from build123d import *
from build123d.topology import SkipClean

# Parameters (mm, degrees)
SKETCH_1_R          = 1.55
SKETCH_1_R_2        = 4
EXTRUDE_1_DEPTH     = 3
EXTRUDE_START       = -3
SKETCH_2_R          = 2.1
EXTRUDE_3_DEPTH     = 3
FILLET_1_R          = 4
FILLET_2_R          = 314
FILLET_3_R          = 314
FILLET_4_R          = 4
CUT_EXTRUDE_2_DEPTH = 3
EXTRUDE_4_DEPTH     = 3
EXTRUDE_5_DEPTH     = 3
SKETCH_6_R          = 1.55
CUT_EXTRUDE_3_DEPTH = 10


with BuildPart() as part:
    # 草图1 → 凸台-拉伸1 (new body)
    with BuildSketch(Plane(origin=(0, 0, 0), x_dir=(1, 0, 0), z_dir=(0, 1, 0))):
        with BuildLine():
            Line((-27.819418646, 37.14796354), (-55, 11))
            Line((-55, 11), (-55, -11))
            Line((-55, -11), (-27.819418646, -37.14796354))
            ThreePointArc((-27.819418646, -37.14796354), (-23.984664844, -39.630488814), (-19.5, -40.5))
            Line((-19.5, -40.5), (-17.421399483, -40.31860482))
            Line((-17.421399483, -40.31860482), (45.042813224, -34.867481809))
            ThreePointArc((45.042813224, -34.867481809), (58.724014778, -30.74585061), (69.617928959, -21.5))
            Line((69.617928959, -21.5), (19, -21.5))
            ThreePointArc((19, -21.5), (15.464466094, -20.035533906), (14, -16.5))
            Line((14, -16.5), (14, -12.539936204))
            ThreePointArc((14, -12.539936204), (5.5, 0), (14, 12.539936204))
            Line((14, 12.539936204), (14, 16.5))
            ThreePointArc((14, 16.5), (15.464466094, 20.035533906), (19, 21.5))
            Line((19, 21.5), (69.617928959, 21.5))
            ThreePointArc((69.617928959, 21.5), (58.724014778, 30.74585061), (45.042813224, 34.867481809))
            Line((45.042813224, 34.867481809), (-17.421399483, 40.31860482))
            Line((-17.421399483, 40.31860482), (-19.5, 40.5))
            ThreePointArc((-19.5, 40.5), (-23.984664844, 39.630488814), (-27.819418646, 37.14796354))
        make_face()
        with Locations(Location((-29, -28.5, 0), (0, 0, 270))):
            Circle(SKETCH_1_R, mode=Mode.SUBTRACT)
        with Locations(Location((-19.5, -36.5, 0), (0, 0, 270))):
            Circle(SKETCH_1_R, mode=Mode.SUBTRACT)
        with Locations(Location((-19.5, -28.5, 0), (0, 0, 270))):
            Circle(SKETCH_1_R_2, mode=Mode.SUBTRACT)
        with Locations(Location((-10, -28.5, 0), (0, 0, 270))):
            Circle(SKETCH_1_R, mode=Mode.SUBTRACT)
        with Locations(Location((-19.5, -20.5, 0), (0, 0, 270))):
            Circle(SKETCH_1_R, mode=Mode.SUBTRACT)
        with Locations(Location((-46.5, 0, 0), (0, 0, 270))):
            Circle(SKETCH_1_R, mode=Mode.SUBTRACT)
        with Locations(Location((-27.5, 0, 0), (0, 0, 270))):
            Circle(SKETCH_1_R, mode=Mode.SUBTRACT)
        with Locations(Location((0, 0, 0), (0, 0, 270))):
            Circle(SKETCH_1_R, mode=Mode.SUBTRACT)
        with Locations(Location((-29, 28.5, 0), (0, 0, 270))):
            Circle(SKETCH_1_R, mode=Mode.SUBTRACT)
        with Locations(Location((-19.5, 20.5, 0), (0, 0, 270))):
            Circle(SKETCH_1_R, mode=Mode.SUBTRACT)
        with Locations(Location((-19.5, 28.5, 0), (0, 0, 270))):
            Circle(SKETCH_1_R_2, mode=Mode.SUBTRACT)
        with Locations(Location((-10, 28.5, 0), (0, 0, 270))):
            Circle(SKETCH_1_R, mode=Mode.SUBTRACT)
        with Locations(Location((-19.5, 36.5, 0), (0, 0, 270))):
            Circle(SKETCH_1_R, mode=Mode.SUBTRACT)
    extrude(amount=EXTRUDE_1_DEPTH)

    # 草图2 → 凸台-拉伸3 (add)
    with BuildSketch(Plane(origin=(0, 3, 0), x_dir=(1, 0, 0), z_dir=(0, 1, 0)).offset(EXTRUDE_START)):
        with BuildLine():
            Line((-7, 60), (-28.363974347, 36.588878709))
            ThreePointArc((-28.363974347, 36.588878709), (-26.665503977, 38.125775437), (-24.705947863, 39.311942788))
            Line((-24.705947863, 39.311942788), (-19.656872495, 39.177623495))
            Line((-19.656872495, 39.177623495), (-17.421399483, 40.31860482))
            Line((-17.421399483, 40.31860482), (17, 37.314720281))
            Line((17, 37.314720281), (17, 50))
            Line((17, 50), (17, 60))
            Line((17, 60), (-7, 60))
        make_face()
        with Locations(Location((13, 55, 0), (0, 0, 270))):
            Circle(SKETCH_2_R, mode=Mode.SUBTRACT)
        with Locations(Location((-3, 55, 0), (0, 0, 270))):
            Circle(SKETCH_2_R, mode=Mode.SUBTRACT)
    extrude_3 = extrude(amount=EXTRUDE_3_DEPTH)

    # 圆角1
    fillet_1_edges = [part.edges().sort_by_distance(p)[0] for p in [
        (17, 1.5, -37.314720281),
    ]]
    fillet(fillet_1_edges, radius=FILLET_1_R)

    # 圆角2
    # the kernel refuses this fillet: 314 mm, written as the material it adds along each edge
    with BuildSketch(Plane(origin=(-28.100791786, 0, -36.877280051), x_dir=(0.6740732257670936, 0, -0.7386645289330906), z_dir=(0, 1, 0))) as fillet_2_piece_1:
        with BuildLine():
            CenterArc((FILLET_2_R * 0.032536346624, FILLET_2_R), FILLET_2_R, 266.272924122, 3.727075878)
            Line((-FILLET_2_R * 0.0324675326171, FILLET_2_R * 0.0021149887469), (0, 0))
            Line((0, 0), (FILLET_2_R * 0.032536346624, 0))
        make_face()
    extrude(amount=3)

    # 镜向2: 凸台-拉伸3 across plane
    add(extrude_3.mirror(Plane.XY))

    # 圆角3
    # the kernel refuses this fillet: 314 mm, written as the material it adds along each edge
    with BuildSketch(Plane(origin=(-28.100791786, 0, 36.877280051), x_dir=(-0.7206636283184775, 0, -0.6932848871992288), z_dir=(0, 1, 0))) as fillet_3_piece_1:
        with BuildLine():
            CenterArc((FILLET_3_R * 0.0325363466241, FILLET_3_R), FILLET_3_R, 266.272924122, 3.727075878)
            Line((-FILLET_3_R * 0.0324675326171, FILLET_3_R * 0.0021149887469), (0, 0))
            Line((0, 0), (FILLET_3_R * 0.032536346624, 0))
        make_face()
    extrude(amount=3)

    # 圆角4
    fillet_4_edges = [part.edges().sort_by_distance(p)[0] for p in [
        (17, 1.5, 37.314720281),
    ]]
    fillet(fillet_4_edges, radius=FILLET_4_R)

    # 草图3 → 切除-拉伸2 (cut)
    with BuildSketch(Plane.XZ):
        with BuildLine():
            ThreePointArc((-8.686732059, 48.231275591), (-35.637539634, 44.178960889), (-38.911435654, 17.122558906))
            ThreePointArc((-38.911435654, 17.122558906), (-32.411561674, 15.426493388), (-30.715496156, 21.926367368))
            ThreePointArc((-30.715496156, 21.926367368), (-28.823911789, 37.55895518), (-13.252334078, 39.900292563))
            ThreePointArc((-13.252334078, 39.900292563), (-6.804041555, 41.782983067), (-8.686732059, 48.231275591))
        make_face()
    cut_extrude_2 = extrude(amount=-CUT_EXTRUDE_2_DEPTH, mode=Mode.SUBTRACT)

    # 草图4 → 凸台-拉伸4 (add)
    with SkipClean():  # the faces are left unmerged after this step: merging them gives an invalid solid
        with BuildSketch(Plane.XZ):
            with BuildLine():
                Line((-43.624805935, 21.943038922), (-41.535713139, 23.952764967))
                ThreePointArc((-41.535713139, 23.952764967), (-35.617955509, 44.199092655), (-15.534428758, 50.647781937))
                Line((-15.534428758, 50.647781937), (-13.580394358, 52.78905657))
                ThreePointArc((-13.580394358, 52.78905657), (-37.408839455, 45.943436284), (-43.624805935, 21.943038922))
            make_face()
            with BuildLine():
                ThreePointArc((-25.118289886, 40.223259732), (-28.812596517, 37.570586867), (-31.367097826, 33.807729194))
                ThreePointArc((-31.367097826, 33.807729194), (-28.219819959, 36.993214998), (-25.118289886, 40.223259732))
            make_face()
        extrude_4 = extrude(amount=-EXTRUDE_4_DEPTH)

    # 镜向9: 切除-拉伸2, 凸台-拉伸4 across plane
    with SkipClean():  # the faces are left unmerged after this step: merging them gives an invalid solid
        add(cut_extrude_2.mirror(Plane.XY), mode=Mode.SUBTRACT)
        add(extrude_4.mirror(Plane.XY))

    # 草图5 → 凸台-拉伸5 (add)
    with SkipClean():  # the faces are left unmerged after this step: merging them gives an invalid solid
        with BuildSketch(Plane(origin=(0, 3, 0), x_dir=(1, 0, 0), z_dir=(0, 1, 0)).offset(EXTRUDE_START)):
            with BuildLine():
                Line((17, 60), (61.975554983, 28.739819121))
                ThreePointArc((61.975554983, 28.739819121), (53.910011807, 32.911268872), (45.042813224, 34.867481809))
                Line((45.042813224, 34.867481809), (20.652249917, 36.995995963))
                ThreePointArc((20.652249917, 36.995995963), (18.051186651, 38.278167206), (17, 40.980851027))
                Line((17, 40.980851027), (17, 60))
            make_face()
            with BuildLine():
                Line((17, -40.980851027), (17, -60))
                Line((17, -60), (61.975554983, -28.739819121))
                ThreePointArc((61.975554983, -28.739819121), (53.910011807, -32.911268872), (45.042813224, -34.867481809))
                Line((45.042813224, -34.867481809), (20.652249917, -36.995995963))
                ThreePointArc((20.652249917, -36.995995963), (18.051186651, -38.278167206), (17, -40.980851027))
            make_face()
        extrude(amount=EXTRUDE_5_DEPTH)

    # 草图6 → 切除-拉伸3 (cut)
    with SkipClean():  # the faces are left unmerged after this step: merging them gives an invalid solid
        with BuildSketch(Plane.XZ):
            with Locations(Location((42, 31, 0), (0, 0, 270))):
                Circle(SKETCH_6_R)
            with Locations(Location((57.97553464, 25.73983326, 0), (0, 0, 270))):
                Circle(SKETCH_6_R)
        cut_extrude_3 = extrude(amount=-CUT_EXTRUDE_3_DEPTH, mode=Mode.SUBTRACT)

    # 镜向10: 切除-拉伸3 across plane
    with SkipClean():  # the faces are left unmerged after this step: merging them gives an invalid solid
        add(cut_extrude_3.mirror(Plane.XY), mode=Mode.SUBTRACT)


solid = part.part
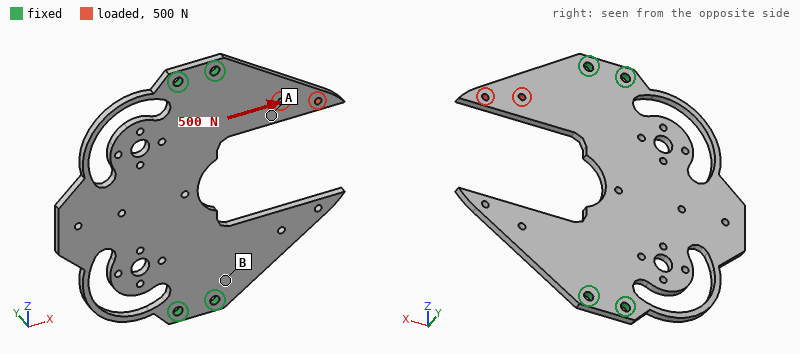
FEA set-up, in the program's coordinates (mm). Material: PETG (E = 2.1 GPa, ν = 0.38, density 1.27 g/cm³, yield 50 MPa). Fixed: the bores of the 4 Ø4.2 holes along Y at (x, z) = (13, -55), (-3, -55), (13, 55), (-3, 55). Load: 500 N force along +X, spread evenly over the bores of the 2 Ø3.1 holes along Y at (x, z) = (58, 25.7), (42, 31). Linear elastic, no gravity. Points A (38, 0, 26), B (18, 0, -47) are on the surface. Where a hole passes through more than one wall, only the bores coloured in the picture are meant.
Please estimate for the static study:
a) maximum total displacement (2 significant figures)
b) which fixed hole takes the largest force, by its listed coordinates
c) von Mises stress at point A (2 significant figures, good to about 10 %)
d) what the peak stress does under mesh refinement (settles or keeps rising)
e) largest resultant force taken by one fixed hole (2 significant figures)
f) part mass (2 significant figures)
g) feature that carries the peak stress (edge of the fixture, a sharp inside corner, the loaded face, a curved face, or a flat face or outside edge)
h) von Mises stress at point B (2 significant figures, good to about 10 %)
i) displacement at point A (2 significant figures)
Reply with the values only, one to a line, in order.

1.1 mm
(13, 55)
13 MPa
keeps rising
350 N
29 g
edge of the fixture
2.4 MPa
0.49 mm
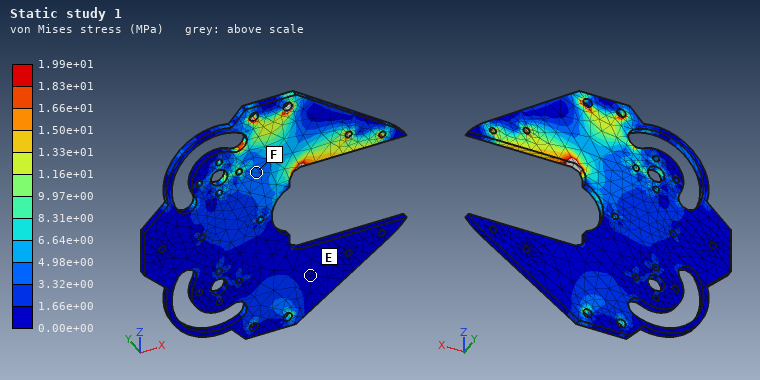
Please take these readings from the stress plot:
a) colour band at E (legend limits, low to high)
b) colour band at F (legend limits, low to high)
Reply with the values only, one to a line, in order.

0.00e+00 to 1.66e+00 MPa
3.32e+00 to 4.98e+00 MPa
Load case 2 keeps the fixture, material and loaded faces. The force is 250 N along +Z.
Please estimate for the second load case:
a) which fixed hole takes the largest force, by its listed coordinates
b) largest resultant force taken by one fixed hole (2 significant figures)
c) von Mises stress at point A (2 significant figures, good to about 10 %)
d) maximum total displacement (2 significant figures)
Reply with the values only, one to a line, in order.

(13, 55)
430 N
7.9 MPa
1.2 mm
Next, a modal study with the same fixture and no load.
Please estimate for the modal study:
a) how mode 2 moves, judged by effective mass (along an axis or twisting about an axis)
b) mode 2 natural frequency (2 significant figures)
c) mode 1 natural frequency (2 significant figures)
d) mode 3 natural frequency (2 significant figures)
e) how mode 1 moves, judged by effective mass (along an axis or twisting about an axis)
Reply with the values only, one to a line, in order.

along Y
260 Hz
160 Hz
270 Hz
along Y
